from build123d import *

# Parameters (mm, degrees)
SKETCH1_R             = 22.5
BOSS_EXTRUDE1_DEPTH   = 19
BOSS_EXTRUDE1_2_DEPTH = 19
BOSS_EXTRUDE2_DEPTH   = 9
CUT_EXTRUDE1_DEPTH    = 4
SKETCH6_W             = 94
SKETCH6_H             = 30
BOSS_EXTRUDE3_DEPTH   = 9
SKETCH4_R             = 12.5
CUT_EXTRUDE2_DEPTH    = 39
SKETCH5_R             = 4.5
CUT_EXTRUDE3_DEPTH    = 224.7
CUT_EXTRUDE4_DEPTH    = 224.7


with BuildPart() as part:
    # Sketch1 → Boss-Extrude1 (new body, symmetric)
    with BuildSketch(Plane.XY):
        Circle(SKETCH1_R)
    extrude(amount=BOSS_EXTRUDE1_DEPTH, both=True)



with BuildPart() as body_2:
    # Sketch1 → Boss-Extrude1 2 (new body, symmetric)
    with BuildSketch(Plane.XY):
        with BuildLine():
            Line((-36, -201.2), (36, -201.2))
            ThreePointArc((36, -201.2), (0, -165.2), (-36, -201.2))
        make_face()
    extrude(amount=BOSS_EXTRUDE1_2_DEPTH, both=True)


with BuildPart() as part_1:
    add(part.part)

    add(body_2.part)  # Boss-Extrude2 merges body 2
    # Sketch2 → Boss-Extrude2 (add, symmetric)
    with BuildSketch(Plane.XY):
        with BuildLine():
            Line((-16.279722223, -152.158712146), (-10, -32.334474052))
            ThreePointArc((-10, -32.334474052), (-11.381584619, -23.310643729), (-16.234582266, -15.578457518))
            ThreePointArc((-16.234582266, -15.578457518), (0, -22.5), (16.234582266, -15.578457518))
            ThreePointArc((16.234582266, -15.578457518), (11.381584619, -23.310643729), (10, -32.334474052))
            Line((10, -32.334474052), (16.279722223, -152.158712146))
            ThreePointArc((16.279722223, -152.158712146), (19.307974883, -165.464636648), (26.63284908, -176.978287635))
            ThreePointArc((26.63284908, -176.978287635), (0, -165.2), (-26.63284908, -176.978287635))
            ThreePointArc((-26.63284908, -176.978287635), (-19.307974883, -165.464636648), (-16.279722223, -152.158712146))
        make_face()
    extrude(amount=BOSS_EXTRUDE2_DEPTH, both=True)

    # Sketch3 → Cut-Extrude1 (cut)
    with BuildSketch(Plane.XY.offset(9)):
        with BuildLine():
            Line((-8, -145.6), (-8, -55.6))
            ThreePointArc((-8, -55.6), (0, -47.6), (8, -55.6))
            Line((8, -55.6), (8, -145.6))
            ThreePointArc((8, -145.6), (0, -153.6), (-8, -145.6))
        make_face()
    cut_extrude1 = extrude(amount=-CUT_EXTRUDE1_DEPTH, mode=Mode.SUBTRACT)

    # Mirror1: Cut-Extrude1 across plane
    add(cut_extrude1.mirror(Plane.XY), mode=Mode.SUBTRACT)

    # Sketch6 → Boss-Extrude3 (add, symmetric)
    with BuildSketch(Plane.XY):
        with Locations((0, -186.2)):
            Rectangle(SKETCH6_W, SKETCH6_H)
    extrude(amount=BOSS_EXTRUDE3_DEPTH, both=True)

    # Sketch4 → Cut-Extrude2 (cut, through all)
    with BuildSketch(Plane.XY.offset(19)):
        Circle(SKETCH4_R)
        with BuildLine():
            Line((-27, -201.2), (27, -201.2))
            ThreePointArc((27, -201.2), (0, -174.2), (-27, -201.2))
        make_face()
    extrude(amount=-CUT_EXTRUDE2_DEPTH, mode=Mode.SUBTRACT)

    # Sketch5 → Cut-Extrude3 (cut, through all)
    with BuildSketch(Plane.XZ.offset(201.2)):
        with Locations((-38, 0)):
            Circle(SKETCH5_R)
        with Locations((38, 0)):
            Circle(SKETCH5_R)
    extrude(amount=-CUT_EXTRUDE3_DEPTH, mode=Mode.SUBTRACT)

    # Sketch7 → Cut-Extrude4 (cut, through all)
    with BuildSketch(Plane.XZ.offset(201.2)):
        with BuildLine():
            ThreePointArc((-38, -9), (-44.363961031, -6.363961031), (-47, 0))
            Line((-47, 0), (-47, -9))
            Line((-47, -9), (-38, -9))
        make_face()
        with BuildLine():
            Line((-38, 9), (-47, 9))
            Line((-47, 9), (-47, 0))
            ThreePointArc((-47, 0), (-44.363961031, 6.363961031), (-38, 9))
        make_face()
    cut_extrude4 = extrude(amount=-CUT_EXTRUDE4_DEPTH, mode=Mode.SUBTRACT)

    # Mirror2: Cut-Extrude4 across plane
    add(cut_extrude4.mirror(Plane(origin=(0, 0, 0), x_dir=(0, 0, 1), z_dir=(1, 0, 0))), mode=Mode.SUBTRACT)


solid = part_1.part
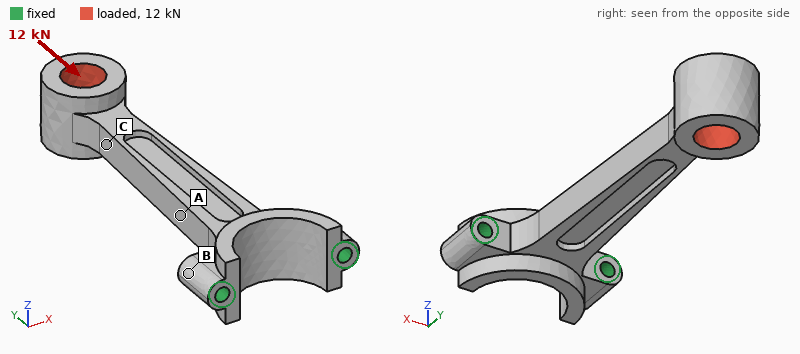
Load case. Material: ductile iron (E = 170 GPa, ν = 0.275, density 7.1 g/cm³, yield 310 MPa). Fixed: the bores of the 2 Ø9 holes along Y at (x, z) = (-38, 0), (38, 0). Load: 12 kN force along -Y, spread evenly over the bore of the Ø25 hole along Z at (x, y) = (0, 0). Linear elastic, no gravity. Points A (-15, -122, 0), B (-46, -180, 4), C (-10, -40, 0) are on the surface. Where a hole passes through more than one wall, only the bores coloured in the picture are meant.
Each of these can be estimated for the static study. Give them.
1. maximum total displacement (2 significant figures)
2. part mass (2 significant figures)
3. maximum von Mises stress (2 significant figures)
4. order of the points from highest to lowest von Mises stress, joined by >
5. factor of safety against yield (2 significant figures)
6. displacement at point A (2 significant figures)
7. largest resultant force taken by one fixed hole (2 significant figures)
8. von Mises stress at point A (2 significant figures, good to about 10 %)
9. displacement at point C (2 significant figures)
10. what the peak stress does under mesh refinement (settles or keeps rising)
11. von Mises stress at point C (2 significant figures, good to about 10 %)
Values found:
43 µm
1.0 kg
68 MPa
C > A > B
4.5
14 µm
7.5 kN
30 MPa
31 µm
settles
38 MPa
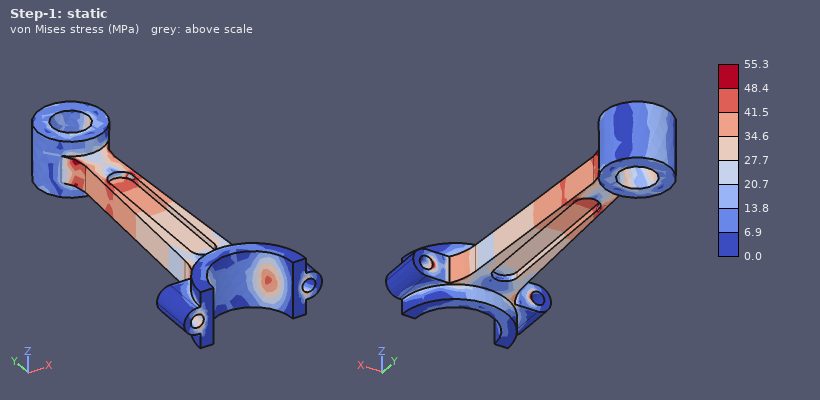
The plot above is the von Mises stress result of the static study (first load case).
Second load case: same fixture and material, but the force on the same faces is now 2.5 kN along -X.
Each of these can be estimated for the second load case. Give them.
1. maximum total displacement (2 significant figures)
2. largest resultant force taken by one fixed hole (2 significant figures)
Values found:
0.99 mm
9.9 kN
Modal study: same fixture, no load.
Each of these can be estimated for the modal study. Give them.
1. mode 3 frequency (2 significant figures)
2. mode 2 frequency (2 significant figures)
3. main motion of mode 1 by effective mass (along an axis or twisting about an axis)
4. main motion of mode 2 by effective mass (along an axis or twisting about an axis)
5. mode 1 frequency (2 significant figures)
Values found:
1200 Hz
470 Hz
along Z
along X
230 Hz
